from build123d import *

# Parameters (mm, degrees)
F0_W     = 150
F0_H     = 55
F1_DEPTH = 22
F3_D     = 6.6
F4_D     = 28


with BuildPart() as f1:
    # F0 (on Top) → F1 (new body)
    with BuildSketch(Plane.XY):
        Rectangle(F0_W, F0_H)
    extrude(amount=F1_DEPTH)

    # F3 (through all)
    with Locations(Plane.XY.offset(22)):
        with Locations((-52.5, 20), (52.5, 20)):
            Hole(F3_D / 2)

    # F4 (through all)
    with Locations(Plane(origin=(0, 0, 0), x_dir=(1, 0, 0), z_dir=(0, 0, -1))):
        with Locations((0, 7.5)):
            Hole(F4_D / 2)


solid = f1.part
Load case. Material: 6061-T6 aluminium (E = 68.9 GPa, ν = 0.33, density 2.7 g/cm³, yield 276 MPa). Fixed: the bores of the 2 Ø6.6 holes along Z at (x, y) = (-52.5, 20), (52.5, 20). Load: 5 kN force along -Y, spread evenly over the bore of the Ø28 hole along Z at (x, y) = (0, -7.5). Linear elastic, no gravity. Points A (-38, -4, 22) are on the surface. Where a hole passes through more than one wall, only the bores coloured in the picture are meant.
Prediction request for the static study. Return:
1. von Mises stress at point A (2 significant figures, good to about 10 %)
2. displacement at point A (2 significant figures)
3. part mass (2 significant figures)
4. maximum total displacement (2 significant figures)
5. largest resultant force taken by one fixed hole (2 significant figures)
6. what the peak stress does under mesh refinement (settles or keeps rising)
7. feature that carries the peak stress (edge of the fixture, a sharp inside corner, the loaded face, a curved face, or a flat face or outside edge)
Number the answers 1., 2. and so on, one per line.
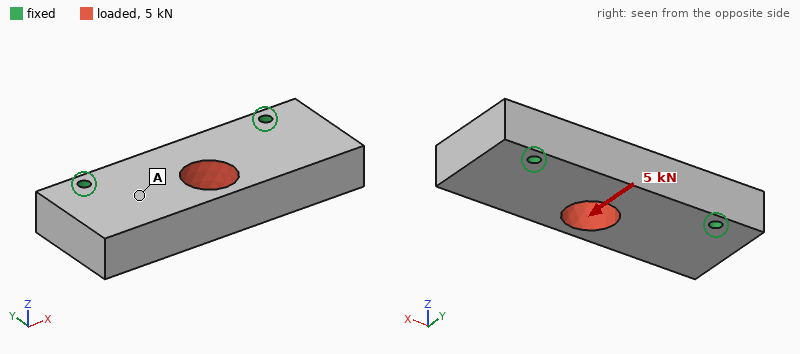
1. 4.7 MPa
2. 4.0 µm
3. 450 g
4. 9.6 µm
5. 3.0 kN
6. keeps rising
7. edge of the fixture
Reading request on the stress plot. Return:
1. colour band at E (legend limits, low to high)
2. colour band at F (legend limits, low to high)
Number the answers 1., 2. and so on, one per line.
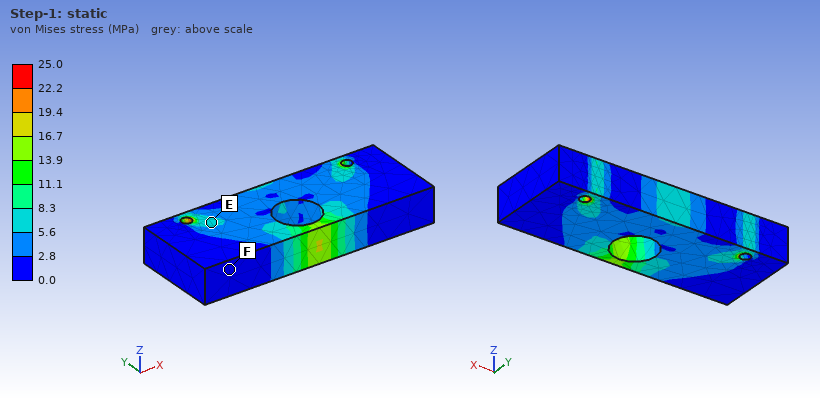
1. 5.6 to 8.3 MPa
2. 0.0 to 2.8 MPa
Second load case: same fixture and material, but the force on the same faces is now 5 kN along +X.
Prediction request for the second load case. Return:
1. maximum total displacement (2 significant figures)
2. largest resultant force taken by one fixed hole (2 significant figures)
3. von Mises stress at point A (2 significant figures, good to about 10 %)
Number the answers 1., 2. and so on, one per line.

1. 6.7 µm
2. 2.8 kN
3. 2.8 MPa
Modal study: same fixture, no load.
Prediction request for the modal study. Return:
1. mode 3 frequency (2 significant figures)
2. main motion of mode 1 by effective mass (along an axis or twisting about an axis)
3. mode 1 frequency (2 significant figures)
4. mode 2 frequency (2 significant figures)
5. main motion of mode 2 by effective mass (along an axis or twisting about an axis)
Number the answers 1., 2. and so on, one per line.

1. 7300 Hz
2. along Z
3. 4200 Hz
4. 6300 Hz
5. twisting about Y
